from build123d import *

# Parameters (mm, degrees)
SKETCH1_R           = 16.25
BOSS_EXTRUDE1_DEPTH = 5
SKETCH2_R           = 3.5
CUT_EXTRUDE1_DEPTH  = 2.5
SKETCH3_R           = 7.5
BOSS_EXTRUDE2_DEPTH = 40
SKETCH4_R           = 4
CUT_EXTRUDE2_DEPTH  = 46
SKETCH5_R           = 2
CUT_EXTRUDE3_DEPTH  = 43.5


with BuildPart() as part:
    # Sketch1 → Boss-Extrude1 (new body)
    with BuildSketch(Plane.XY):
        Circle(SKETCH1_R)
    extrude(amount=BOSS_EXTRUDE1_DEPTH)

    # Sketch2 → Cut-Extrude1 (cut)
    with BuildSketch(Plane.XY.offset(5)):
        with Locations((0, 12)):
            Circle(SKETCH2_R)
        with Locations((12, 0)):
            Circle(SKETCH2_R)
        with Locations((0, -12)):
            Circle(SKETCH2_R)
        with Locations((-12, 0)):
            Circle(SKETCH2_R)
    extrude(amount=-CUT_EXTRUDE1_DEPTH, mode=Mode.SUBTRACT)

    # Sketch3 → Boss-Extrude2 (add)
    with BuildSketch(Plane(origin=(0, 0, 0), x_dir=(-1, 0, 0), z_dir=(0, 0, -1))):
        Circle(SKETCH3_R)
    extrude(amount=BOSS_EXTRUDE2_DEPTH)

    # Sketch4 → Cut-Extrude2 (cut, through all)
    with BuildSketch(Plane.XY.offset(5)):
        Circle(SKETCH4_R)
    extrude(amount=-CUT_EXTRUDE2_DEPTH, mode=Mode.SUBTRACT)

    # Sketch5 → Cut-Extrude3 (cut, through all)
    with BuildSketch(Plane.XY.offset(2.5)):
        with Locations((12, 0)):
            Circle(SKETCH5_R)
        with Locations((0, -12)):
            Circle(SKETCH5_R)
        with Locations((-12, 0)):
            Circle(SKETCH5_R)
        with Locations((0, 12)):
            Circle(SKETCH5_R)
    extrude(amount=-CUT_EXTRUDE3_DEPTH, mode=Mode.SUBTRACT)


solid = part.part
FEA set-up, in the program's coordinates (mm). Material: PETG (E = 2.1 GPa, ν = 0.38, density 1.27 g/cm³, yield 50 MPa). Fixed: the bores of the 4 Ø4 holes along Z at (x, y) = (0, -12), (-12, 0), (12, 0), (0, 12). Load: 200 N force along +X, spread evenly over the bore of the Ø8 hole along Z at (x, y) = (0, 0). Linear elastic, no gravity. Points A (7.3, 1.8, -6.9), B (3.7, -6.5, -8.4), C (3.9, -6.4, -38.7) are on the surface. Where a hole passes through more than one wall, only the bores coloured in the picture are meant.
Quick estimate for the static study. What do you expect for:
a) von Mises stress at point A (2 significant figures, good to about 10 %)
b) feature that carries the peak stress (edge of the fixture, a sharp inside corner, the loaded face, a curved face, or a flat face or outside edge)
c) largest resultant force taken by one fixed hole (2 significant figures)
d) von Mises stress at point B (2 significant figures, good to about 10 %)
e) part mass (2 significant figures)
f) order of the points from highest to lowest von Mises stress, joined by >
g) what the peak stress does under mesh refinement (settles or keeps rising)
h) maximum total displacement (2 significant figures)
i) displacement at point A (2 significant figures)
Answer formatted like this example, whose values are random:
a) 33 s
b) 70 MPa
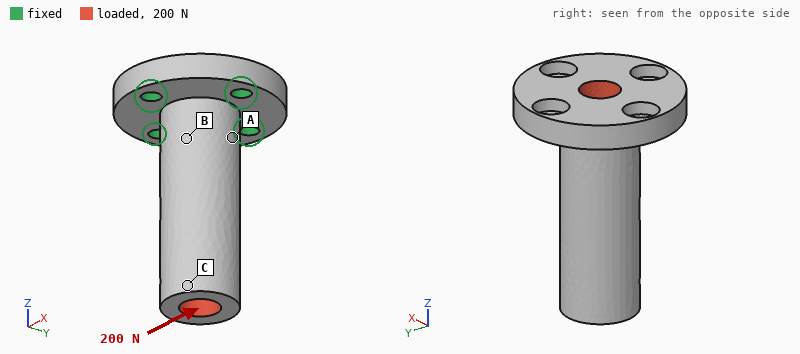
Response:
a) 7.4 MPa
b) edge of the fixture
c) 170 N
d) 4.2 MPa
e) 11 g
f) A > B > C
g) keeps rising
h) 0.63 mm
i) 0.12 mm
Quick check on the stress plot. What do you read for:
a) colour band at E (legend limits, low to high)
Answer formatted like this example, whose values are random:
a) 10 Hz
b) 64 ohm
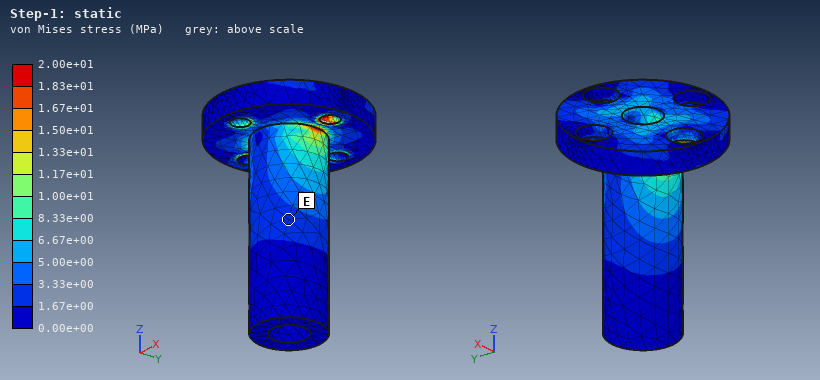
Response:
a) 1.67e+00 to 3.33e+00 MPa
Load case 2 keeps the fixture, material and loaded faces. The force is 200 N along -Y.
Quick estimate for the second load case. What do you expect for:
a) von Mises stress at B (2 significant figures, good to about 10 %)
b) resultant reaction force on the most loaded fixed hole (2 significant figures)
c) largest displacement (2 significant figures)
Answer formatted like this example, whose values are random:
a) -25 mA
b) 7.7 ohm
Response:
a) 6.2 MPa
b) 170 N
c) 0.63 mm
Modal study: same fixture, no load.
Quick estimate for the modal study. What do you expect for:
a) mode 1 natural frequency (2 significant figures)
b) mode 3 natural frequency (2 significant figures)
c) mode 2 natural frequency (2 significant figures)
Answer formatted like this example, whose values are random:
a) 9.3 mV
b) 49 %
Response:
a) 1300 Hz
b) 4600 Hz
c) 1300 Hz
